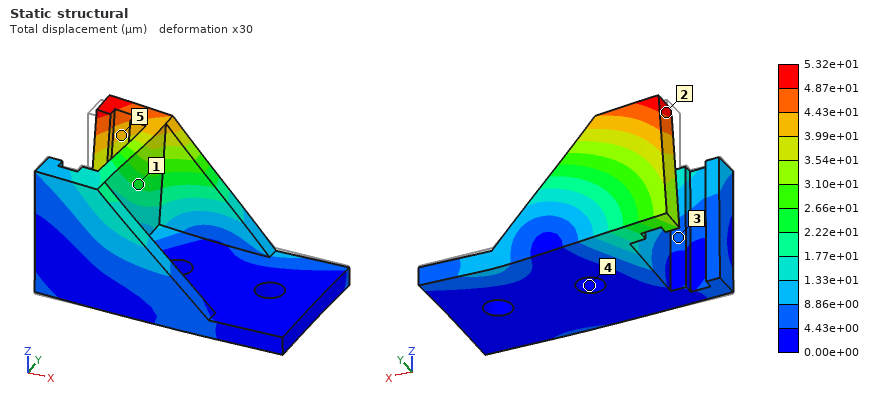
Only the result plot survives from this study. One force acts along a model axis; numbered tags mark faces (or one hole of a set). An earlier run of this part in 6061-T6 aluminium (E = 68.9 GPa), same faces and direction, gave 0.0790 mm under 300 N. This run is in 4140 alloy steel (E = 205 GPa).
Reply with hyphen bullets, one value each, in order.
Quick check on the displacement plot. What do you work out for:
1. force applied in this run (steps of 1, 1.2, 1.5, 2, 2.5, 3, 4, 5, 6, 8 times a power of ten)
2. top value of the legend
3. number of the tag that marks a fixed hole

- 600 N
- 5.32e+01 µm
- 4
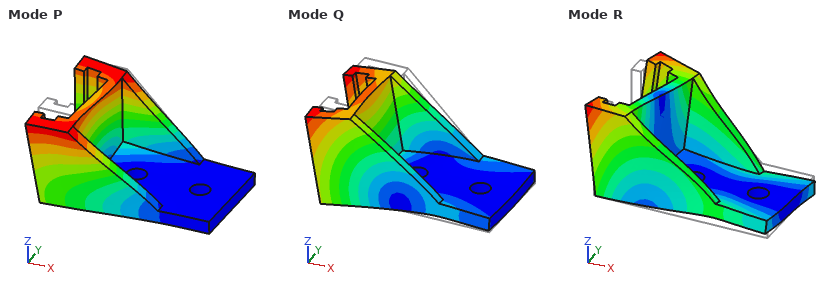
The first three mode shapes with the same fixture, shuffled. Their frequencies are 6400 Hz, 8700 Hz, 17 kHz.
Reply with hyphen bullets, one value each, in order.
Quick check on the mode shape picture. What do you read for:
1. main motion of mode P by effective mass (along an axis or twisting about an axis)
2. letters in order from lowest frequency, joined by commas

- along Y
- P, Q, R
